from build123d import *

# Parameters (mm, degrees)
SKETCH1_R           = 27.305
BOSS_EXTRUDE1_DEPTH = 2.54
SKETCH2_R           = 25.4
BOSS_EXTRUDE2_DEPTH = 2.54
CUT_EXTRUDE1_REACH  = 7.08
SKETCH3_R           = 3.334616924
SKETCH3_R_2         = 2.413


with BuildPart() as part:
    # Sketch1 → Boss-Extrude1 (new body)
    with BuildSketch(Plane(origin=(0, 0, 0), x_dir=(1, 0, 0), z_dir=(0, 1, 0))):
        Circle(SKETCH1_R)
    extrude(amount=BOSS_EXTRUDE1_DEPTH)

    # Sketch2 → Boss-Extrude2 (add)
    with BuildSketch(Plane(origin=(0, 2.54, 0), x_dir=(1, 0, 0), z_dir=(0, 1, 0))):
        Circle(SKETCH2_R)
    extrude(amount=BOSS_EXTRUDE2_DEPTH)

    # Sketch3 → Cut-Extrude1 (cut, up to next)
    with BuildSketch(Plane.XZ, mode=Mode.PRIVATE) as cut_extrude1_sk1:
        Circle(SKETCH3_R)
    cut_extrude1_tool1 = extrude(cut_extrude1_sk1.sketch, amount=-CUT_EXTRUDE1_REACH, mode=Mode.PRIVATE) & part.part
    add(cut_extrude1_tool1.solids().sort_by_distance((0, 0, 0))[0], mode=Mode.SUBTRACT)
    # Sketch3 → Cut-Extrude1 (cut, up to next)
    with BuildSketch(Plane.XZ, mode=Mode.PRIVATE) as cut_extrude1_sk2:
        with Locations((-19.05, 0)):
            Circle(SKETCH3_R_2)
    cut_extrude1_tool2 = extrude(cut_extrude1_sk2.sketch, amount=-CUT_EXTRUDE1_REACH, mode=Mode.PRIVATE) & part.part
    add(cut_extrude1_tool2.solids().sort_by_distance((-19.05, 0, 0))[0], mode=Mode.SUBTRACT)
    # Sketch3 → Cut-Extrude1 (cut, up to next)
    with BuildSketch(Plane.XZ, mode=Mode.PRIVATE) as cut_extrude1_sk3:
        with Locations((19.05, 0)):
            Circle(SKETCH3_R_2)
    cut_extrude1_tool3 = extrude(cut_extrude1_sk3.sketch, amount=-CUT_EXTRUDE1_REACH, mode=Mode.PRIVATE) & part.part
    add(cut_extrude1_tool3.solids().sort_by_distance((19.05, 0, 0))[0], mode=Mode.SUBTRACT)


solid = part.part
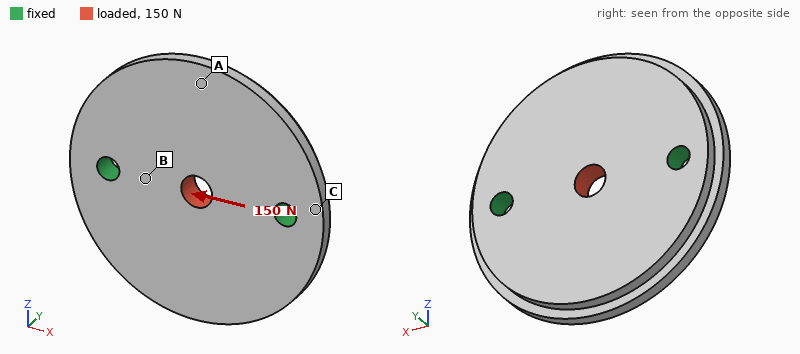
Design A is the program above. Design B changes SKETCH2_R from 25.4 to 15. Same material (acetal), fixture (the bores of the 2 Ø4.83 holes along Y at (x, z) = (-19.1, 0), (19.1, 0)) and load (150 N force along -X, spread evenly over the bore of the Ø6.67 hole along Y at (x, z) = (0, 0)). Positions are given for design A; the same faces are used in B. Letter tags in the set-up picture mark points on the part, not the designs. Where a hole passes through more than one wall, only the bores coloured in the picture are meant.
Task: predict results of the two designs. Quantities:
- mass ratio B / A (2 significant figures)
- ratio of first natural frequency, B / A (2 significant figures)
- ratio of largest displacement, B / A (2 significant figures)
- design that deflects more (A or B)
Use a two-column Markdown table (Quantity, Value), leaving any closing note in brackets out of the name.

| Quantity | Value |
|---|---|
| mass ratio B / A | 0.70 |
| ratio of first natural frequency, B / A | 0.63 |
| ratio of largest displacement, B / A | 1.4 |
| design that deflects more | B |
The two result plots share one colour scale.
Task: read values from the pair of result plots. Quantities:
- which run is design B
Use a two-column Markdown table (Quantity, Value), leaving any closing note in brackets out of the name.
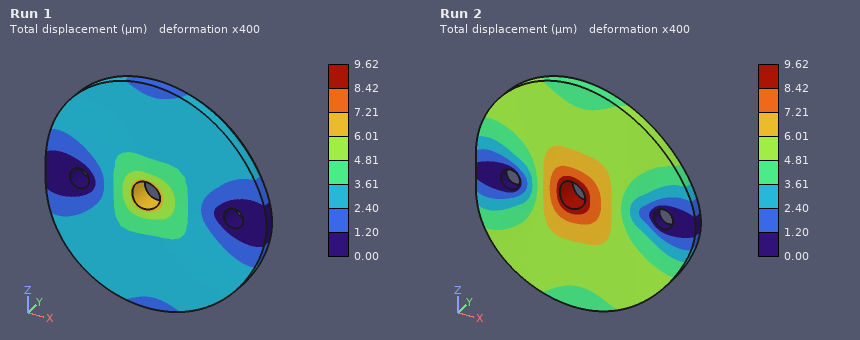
| Quantity | Value |
|---|---|
| which run is design B | Run 2 |
